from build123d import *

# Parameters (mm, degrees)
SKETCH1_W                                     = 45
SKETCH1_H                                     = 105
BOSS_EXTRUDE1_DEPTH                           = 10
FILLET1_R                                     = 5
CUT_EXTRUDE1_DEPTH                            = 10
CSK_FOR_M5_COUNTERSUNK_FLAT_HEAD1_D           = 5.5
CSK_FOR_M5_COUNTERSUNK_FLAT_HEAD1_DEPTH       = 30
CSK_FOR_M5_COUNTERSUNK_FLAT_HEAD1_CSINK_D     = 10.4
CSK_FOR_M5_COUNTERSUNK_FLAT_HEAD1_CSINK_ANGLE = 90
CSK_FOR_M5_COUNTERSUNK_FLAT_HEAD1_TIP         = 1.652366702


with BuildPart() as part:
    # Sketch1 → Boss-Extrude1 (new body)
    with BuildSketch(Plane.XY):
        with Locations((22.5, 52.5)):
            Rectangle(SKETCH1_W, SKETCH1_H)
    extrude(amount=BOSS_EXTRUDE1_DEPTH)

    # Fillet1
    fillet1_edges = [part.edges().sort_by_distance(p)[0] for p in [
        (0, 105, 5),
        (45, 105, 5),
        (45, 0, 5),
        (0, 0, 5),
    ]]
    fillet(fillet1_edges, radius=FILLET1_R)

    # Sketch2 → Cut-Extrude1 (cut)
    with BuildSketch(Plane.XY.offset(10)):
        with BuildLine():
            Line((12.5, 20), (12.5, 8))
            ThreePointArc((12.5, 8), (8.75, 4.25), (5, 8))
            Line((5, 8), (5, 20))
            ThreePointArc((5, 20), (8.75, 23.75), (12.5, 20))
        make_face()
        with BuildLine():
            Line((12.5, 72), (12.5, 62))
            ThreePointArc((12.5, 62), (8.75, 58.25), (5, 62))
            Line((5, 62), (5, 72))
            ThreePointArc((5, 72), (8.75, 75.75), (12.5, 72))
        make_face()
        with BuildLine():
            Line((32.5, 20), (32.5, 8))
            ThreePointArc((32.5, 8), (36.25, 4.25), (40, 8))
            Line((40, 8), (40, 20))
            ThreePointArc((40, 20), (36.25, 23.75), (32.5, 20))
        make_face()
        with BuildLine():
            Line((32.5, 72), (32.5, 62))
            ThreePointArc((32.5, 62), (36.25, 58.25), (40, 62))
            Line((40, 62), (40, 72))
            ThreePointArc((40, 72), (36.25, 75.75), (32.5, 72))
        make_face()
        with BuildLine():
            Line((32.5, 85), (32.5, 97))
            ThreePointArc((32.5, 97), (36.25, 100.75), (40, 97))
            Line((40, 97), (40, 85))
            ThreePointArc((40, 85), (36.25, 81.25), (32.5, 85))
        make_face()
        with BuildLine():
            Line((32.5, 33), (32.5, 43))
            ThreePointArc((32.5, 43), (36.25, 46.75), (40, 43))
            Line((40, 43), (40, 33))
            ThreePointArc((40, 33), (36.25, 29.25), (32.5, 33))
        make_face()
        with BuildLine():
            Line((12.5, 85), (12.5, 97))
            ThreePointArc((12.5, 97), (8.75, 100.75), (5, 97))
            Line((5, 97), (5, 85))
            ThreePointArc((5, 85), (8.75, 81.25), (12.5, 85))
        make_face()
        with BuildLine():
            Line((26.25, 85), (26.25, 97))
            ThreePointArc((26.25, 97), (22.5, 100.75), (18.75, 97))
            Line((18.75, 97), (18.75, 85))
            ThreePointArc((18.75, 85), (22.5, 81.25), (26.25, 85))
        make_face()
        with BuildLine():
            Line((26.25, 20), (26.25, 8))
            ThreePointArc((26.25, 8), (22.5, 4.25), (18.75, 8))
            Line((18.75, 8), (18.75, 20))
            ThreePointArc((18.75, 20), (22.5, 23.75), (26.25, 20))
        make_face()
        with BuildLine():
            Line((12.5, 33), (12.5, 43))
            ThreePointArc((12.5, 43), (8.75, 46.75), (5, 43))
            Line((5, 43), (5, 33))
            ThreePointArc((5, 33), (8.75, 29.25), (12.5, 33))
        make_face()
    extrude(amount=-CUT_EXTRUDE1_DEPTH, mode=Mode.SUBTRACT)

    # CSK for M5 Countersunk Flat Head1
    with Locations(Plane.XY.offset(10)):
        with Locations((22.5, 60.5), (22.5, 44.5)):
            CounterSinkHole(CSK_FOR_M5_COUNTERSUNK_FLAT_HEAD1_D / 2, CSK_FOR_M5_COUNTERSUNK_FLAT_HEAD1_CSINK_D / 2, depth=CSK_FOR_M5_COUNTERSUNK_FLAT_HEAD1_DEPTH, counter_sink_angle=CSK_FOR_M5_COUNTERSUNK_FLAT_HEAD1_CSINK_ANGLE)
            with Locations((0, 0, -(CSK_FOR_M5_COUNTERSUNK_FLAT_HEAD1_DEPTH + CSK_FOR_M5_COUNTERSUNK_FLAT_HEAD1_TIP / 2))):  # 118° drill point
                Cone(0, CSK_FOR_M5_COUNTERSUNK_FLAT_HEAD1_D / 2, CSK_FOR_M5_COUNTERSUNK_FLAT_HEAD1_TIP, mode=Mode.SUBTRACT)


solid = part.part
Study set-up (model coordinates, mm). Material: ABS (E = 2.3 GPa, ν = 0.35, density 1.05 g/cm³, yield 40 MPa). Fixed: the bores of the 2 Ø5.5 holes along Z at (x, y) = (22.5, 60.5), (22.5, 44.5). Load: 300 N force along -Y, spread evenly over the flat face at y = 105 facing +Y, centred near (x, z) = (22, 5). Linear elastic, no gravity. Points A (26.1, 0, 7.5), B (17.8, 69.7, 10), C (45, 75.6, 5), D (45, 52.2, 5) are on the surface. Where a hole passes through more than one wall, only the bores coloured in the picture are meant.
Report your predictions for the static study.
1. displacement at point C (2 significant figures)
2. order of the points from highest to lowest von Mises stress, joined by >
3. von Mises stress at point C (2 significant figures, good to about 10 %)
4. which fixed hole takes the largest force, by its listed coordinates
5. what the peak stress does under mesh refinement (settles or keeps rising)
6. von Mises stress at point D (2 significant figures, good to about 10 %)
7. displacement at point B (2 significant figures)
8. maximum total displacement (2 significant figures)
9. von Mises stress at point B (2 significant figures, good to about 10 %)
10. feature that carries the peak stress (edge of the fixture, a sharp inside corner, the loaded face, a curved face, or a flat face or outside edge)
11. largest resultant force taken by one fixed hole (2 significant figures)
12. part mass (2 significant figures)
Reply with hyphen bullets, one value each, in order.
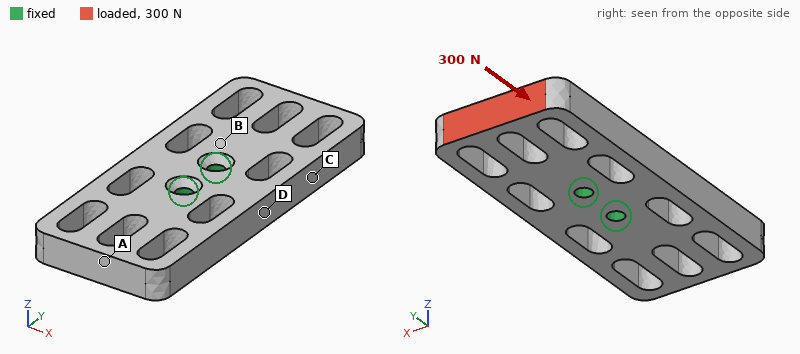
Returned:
- 14 µm
- B > C > D > A
- 0.89 MPa
- (22.5, 60.5)
- keeps rising
- 0.47 MPa
- 8.3 µm
- 36 µm
- 1.1 MPa
- edge of the fixture
- 220 N
- 35 g
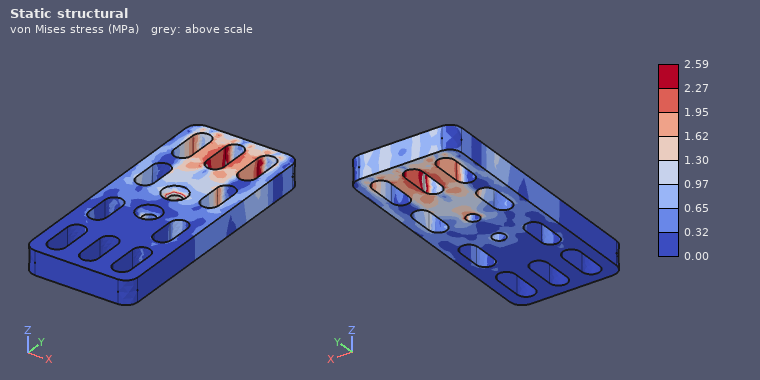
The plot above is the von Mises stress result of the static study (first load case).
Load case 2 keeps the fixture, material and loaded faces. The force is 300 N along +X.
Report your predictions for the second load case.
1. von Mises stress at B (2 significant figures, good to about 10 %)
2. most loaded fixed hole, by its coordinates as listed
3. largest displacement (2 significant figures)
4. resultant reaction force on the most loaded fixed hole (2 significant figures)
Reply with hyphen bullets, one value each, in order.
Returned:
- 3.3 MPa
- (22.5, 60.5)
- 0.50 mm
- 890 N
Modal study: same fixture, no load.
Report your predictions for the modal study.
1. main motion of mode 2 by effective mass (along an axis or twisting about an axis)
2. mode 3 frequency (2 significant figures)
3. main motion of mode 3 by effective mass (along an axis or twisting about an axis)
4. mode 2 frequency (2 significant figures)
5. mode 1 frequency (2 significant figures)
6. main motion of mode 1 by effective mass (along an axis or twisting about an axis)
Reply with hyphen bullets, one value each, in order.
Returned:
- along Z
- 1500 Hz
- twisting about Z
- 1000 Hz
- 990 Hz
- twisting about X
